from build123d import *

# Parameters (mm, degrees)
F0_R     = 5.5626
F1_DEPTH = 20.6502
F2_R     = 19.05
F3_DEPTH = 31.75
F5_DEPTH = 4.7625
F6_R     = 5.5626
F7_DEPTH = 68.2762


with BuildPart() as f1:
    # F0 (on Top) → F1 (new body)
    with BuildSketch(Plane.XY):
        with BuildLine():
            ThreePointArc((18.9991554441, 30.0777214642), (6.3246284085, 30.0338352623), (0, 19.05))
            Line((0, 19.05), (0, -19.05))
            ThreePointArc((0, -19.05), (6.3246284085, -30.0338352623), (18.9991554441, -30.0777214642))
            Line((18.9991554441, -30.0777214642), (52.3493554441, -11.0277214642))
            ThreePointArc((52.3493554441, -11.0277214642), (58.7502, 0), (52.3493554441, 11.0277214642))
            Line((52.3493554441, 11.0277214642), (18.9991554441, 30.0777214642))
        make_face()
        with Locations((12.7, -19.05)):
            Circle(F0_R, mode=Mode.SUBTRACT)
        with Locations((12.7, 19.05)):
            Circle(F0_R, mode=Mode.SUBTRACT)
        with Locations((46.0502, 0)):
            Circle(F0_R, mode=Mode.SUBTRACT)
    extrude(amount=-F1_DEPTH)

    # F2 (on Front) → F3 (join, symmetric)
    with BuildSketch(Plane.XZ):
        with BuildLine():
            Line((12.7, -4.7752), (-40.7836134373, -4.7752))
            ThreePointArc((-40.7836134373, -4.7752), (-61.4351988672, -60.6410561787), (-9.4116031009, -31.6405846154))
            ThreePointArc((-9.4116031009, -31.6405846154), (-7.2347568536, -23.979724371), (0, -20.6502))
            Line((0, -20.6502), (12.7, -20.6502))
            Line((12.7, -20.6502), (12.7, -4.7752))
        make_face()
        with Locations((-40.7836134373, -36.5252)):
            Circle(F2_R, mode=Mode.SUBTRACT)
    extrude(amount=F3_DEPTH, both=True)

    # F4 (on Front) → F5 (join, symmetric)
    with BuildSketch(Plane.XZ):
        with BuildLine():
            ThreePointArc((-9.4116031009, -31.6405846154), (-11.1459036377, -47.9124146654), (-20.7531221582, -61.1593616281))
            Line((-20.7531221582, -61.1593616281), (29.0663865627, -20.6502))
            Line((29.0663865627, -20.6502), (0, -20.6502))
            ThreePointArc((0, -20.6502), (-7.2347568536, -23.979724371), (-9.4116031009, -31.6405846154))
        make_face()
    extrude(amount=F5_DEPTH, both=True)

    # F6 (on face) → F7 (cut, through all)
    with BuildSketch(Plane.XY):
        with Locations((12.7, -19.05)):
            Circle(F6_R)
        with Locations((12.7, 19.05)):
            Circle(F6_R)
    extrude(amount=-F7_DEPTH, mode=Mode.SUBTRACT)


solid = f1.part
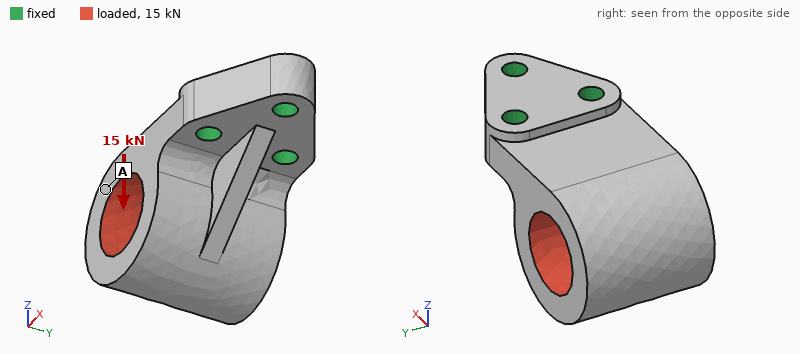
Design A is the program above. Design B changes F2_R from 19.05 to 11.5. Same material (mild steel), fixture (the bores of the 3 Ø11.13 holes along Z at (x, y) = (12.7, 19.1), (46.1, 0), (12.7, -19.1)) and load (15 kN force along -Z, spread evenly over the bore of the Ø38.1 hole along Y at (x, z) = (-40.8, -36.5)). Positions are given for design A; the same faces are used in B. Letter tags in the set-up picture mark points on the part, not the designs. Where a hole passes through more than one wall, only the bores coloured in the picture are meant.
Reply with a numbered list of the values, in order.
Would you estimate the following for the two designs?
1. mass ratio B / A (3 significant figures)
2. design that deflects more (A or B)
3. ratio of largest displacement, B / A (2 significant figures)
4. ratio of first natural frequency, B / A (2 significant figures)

1. 1.22
2. A
3. 0.90
4. 0.92
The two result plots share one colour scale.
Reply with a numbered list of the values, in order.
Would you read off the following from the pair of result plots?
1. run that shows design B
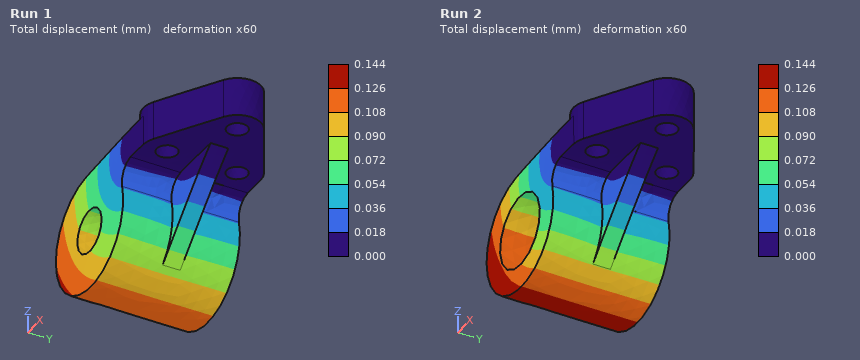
1. Run 1
